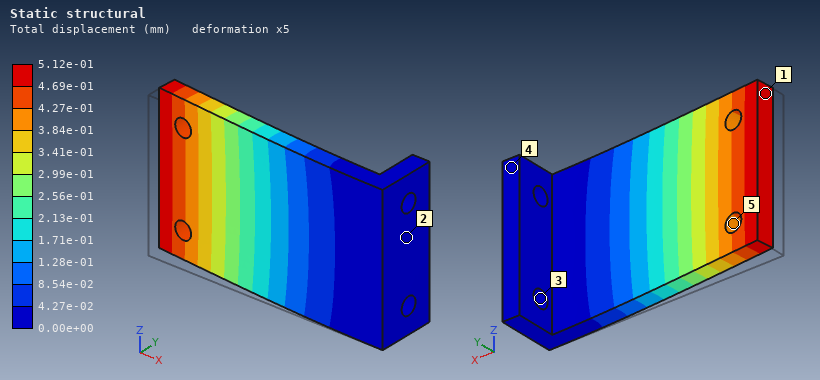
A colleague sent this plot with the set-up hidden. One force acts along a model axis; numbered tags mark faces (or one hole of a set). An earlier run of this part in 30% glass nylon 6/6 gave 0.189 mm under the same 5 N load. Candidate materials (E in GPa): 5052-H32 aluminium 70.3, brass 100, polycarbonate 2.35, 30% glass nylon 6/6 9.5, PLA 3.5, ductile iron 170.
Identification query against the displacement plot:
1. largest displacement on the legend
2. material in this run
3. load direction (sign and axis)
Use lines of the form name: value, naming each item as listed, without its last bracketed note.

largest displacement on the legend: 5.12e-01 mm
material in this run: PLA
load direction: +Y
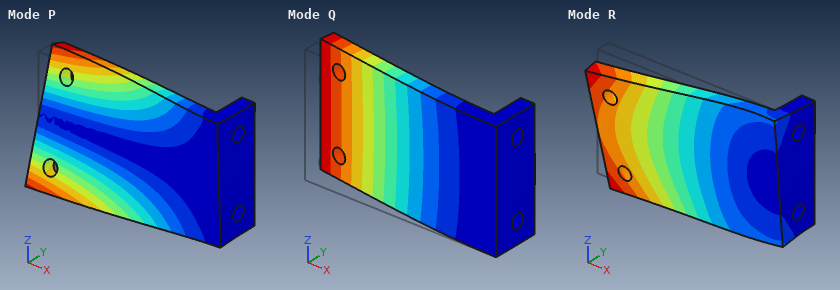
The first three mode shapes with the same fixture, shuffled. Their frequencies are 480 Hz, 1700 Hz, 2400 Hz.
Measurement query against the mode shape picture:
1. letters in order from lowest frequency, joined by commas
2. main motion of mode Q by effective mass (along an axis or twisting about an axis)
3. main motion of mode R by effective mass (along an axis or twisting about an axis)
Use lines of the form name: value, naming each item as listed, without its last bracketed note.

letters in order from lowest frequency, joined by commas: Q, P, R
main motion of mode Q by effective mass: along Y
main motion of mode R by effective mass: along Z
